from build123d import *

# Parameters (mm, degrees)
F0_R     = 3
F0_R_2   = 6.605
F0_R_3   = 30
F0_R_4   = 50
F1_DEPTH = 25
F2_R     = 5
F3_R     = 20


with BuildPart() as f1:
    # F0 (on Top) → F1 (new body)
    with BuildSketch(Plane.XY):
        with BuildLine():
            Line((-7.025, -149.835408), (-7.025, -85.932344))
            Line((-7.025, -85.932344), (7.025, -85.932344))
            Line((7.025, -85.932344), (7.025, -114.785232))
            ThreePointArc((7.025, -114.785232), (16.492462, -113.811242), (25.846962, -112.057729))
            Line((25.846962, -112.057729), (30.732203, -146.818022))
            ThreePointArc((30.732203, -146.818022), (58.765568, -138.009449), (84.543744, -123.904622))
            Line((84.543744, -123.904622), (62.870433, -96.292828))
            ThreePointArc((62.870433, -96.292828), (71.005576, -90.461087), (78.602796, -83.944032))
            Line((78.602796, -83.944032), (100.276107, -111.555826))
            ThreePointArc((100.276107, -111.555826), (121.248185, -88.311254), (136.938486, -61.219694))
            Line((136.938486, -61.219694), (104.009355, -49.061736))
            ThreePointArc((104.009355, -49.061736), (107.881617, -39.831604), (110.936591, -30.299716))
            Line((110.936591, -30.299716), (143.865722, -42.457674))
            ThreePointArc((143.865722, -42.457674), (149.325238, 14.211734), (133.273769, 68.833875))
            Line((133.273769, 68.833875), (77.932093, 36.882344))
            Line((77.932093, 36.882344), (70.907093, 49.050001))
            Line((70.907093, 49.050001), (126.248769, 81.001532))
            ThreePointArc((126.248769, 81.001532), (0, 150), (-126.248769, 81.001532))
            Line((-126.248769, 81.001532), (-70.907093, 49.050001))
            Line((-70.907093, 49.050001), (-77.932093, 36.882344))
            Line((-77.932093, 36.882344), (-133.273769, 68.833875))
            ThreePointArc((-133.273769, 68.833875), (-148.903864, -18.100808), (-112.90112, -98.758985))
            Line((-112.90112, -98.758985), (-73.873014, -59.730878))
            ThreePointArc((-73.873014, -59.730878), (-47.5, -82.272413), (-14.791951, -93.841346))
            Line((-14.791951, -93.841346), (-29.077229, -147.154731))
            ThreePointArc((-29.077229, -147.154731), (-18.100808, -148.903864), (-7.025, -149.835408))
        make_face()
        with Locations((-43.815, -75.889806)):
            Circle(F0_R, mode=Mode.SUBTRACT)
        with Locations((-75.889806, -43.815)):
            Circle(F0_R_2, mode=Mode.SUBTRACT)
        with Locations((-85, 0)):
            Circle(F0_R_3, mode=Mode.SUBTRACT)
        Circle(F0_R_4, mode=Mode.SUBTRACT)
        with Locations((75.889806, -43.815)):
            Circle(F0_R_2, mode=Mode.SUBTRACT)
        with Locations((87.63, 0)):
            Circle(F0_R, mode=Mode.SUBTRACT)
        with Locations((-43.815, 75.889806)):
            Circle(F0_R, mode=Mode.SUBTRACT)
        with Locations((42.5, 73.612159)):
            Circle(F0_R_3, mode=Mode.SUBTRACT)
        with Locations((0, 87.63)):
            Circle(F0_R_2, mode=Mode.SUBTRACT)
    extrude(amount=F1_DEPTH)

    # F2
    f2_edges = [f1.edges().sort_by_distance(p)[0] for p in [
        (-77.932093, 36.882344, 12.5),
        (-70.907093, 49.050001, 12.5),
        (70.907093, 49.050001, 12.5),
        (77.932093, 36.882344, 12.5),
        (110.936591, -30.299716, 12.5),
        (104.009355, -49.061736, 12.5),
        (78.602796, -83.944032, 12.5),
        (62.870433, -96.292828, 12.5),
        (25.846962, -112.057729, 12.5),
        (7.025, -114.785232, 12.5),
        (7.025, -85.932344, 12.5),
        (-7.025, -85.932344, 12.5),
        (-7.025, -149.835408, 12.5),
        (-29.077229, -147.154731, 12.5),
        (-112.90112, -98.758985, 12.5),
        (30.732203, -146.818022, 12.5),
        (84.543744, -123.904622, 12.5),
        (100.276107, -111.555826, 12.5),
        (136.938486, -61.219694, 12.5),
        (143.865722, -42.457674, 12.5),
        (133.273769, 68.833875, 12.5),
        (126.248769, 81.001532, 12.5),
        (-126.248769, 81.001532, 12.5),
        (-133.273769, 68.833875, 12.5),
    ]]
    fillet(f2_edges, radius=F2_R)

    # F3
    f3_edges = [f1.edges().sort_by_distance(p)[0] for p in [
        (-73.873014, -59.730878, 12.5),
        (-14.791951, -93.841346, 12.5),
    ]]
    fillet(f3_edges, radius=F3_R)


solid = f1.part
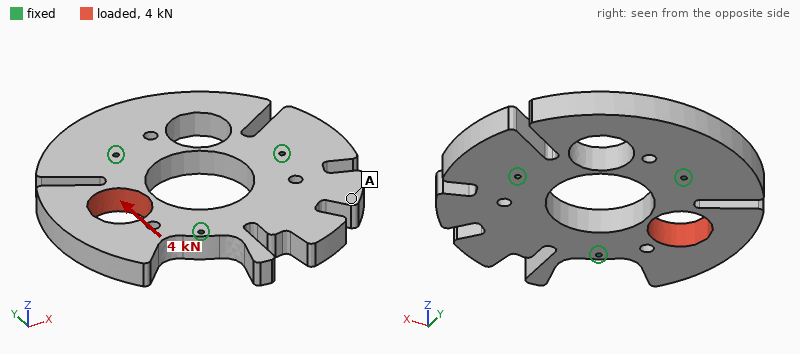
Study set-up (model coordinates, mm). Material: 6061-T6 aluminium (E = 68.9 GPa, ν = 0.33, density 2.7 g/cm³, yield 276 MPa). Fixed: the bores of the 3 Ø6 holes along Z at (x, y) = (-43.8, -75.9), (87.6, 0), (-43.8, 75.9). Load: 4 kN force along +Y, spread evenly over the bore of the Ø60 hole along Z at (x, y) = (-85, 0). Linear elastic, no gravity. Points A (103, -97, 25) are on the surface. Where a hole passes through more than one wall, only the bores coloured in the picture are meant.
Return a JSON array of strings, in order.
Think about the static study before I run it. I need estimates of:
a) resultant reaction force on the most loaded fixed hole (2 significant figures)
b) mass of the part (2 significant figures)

["2.3 kN", "3.2 kg"]
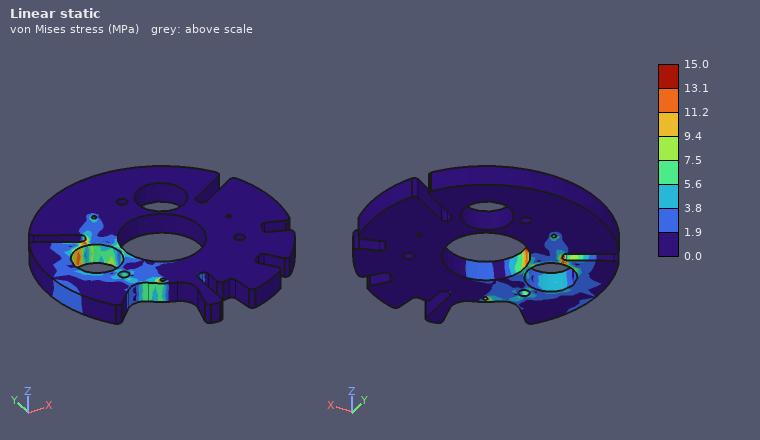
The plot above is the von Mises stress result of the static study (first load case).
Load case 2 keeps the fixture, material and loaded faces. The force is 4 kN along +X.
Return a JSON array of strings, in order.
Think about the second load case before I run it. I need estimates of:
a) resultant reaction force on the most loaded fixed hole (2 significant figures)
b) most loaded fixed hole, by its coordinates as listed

["2.2 kN", "(-43.8, 75.9)"]
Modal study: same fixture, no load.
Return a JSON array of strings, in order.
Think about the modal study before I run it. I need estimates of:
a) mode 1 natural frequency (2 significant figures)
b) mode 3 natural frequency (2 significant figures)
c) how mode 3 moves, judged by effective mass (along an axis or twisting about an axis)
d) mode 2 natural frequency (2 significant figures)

["1000 Hz", "1400 Hz", "along Z", "1200 Hz"]
